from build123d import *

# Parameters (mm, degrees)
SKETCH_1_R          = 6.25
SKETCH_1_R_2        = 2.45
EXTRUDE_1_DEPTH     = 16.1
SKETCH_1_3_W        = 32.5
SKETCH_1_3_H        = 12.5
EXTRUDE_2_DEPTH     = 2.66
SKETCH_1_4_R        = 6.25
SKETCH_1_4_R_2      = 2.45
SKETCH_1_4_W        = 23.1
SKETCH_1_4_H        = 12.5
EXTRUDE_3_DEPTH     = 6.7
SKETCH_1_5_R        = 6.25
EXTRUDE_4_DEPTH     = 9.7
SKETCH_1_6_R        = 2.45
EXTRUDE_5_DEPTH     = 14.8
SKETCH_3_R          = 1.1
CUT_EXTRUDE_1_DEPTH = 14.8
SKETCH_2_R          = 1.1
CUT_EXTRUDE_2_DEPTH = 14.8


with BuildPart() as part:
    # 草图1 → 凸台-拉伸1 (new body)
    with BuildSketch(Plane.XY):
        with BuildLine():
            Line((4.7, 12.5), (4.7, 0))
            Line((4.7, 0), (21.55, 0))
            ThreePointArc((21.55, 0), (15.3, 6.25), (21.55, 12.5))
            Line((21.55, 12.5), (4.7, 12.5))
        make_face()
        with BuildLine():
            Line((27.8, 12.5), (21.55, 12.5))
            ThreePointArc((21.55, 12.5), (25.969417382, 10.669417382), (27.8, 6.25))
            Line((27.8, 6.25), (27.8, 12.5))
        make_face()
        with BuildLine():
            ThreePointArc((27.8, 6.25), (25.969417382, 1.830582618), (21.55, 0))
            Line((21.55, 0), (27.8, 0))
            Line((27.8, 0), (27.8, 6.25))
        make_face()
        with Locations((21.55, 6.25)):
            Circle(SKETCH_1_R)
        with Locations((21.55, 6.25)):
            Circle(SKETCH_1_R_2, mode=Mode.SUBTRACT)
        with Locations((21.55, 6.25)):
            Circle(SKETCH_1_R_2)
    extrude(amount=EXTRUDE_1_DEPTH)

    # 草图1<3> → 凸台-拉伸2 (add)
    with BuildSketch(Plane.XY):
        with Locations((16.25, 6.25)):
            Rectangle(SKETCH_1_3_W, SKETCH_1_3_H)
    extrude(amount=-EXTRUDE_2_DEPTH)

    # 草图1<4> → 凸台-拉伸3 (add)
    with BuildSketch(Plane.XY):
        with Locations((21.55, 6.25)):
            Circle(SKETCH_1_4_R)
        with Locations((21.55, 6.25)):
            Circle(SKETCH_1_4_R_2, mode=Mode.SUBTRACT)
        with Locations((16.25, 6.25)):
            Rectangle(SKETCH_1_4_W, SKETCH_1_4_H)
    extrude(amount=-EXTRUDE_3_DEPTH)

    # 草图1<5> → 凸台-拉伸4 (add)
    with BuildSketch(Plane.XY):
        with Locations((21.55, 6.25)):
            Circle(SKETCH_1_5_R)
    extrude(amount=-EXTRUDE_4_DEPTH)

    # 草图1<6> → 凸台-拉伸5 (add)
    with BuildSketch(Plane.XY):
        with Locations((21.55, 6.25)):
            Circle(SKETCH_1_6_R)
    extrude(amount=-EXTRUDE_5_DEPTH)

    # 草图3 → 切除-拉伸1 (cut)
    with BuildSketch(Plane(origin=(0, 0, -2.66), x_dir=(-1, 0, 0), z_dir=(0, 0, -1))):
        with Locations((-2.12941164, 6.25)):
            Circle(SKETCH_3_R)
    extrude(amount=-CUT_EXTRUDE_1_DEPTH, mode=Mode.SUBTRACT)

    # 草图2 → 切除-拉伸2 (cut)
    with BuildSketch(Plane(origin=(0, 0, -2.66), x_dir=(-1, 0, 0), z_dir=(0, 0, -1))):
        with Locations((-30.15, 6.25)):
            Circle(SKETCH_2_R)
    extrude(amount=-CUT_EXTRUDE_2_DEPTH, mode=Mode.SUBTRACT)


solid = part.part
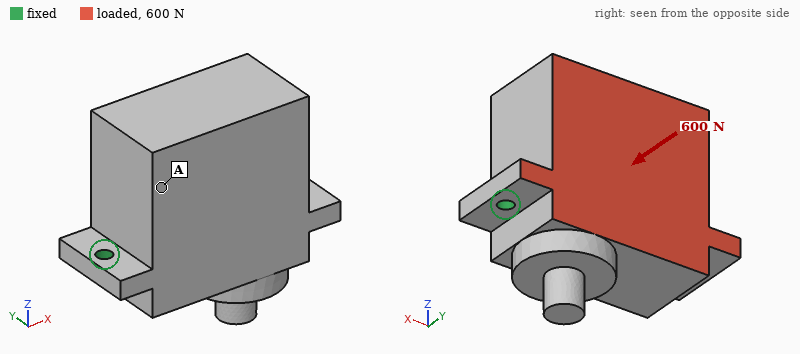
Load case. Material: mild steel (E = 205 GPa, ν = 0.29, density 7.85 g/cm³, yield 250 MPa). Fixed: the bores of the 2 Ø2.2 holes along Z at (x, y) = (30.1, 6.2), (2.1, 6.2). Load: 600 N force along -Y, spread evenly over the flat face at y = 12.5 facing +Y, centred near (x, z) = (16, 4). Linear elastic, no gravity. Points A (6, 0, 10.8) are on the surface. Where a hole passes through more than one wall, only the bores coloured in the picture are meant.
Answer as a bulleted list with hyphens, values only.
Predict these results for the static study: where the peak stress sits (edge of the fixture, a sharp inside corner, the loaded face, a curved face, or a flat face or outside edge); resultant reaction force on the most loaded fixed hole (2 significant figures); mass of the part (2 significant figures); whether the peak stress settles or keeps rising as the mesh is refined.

- edge of the fixture
- 300 N
- 58 g
- keeps rising
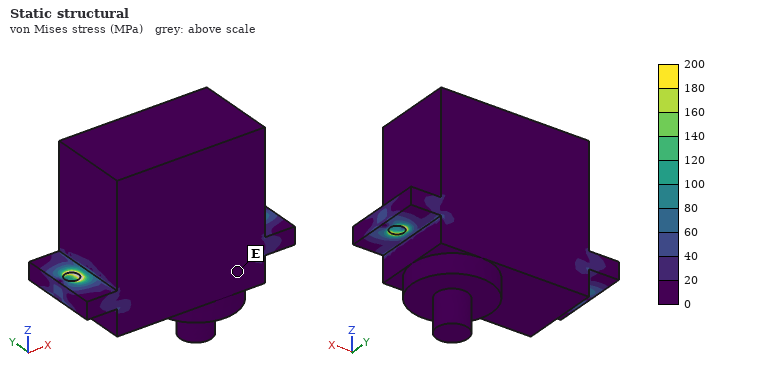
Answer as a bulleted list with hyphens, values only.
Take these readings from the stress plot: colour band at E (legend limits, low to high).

- 0 to 20 MPa
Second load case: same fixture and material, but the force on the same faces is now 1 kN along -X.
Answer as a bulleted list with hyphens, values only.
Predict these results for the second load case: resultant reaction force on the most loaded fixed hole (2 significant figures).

- 600 N
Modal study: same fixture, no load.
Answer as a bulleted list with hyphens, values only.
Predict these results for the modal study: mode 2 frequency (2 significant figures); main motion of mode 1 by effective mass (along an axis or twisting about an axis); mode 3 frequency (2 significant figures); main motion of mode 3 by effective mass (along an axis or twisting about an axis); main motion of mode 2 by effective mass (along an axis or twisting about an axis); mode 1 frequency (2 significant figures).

- 16 kHz
- along Y
- 17 kHz
- along X
- along Z
- 4200 Hz
